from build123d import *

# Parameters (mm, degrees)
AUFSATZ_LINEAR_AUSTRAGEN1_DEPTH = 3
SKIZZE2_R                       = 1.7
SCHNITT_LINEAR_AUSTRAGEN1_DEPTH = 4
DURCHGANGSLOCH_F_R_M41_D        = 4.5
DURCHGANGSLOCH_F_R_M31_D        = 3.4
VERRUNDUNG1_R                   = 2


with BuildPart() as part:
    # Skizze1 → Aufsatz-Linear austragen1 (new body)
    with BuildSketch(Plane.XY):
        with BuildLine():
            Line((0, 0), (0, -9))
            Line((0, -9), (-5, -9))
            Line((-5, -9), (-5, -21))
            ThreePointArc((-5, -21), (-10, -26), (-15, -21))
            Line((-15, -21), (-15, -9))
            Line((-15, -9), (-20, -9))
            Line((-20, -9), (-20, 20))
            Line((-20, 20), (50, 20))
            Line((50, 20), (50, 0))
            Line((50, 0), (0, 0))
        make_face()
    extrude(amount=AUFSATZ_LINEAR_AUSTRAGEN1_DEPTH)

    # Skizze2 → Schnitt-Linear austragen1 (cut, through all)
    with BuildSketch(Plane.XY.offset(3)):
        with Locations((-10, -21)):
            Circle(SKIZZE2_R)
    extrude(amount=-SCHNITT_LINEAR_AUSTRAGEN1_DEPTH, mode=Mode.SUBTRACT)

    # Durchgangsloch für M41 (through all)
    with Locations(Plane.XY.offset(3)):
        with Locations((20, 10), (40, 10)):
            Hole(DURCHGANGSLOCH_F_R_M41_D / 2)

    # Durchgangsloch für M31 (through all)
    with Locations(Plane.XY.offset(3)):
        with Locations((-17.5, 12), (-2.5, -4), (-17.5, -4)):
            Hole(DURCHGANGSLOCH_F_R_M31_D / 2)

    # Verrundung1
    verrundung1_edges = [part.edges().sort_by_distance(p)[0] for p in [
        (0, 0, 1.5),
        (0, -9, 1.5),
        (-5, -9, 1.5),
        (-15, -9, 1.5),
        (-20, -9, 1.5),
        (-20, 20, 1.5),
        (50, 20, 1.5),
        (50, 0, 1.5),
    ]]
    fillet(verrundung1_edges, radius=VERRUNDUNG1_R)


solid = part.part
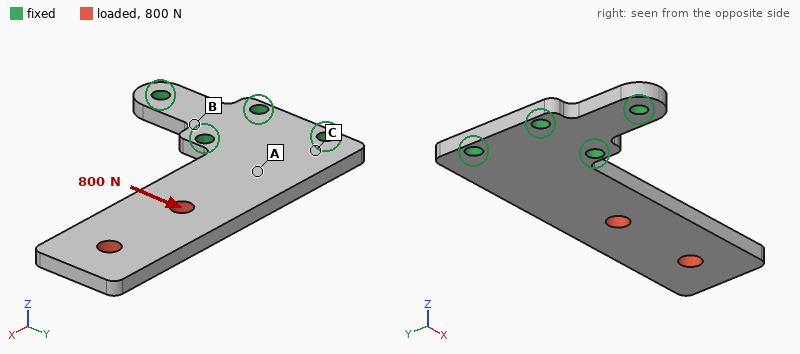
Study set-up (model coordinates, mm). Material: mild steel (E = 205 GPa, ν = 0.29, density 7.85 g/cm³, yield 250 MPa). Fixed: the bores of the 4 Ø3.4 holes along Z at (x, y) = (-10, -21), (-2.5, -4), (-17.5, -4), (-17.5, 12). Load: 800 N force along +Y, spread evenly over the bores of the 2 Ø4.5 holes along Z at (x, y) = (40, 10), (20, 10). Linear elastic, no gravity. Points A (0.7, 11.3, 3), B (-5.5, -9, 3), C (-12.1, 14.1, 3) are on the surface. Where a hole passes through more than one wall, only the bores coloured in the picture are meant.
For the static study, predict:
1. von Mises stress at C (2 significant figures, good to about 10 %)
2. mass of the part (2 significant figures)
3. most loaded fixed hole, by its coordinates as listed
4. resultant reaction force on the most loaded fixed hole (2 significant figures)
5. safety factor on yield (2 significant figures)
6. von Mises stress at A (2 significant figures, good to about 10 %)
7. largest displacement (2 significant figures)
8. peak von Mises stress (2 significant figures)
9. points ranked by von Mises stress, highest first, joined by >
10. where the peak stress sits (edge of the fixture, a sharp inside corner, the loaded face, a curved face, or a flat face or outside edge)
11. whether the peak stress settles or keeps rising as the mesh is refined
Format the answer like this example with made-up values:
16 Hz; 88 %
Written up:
64 MPa; 39 g; (-2.5, -4); 1.5 kN; 0.70; 34 MPa; 75 µm; 360 MPa; C > A > B; a curved face; settles
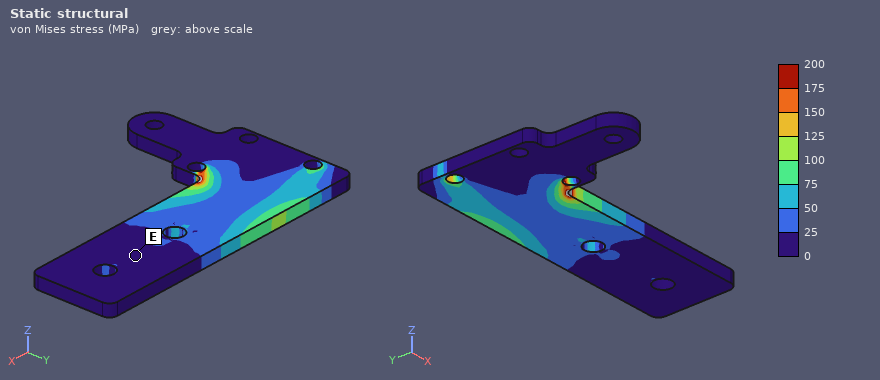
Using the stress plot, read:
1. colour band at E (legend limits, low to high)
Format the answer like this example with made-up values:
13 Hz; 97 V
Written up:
0 to 25 MPa
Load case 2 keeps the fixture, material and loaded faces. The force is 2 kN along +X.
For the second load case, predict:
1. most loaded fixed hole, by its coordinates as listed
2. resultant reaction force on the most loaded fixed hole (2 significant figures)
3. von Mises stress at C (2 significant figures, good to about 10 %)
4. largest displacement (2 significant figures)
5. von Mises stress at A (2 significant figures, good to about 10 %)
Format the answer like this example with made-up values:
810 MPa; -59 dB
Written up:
(-17.5, 12); 1.4 kN; 49 MPa; 13 µm; 33 MPa
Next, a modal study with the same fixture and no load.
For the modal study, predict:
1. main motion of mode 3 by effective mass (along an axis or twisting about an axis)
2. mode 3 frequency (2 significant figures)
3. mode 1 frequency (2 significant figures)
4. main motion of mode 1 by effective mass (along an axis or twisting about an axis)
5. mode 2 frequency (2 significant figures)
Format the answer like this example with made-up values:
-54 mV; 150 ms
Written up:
along Y; 4600 Hz; 740 Hz; along Z; 3600 Hz
